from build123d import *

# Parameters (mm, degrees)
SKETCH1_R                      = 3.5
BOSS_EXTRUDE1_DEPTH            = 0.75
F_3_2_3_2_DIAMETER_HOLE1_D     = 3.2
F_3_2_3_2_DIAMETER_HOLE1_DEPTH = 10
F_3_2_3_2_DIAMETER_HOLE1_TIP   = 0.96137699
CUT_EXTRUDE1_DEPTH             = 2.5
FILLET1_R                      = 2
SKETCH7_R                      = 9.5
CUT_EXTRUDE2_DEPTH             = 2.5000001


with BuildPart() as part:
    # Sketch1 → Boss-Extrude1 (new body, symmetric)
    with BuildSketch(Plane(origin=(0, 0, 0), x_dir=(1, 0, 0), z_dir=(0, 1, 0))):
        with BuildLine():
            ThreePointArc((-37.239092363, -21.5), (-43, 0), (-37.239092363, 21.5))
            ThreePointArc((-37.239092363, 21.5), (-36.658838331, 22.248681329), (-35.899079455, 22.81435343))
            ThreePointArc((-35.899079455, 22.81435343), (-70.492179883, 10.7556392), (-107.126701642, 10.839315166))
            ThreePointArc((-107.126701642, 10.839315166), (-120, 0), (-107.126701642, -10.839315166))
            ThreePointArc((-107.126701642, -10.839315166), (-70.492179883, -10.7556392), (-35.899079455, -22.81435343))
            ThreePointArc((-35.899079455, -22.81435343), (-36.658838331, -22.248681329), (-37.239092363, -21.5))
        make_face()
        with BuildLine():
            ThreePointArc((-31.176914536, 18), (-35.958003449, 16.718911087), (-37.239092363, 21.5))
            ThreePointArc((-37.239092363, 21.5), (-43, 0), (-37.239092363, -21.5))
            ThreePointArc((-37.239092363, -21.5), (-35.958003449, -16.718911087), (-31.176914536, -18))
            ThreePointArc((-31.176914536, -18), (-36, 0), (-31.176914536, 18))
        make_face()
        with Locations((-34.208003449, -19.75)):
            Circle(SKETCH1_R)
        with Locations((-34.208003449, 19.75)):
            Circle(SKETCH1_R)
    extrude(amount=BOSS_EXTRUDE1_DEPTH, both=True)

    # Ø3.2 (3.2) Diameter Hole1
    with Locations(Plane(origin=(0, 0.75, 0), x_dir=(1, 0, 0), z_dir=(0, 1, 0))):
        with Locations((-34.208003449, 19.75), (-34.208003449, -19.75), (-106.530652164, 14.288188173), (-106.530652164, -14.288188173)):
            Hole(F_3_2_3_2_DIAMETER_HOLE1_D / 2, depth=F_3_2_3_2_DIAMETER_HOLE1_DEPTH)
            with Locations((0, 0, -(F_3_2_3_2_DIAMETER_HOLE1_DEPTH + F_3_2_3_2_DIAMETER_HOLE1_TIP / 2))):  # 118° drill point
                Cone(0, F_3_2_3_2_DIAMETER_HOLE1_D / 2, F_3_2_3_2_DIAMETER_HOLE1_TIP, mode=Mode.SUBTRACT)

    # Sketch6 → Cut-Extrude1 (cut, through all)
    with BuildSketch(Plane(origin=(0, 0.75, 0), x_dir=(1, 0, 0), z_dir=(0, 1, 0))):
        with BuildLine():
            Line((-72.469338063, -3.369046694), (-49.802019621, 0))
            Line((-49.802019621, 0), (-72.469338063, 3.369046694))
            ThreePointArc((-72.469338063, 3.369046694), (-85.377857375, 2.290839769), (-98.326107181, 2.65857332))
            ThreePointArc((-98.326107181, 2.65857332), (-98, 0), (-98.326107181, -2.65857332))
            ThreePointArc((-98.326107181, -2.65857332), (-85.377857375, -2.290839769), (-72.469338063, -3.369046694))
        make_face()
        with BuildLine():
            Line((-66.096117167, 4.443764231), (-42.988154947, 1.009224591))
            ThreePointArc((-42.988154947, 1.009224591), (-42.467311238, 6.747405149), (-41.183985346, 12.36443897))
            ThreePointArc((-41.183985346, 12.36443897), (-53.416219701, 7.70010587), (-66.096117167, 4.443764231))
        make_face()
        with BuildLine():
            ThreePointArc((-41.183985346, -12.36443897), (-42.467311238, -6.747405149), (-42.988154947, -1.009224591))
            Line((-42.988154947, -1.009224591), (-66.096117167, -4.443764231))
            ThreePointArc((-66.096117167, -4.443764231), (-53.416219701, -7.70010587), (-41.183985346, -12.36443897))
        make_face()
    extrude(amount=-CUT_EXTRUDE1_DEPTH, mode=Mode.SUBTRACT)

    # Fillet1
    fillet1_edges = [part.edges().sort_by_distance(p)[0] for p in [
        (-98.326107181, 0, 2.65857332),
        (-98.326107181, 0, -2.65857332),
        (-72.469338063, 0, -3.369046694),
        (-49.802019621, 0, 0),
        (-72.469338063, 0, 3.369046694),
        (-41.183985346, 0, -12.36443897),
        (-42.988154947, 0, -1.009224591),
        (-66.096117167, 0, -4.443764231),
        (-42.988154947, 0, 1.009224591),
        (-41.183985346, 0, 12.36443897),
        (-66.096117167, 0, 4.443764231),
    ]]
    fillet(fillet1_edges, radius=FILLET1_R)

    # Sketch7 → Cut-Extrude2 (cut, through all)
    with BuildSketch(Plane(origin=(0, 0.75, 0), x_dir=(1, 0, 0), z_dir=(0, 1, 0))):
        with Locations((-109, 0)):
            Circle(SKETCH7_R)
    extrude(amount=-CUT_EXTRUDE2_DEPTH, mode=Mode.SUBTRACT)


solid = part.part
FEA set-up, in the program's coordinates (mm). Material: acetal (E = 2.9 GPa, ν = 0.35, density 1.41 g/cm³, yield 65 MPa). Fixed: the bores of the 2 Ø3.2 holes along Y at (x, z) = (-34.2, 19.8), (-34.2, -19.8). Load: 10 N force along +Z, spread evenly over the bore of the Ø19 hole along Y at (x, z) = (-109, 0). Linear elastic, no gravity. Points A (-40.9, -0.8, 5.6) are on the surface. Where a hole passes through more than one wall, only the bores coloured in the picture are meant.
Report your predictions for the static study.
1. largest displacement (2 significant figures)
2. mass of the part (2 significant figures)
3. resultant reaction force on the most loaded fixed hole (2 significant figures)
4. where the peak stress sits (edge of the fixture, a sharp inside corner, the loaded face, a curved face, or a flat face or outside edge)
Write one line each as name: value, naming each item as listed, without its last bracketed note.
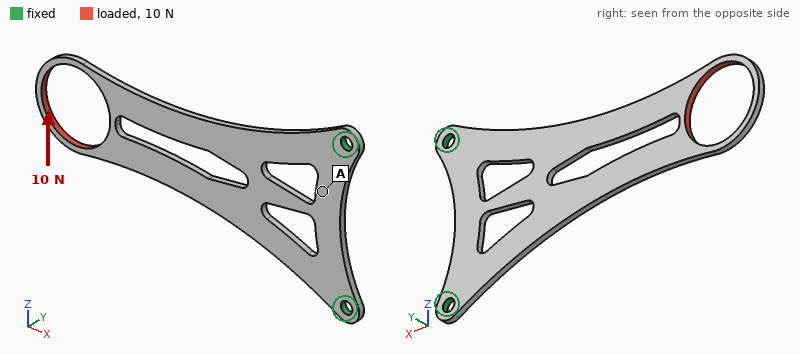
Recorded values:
largest displacement: 1.0 mm
mass of the part: 3.1 g
resultant reaction force on the most loaded fixed hole: 21 N
where the peak stress sits: a curved face
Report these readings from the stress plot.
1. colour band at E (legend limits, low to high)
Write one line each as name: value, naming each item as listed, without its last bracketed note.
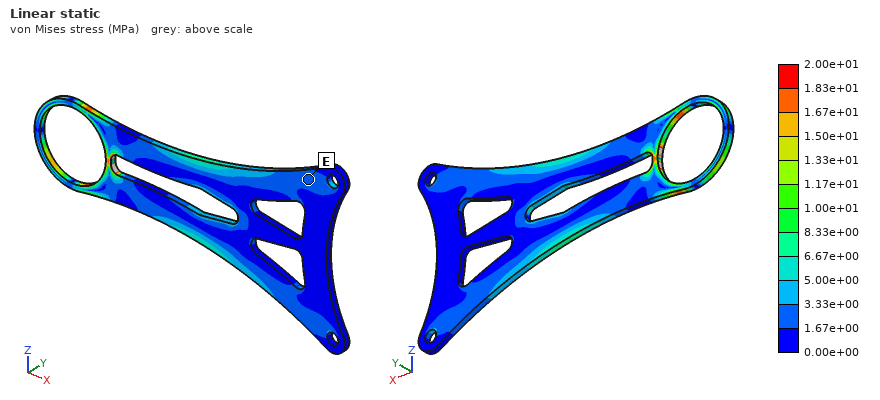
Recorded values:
colour band at E: 1.67e+00 to 3.33e+00 MPa
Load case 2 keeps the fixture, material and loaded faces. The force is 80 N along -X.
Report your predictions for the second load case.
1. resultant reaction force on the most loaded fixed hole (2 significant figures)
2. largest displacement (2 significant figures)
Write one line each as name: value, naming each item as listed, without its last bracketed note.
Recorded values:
resultant reaction force on the most loaded fixed hole: 47 N
largest displacement: 0.72 mm
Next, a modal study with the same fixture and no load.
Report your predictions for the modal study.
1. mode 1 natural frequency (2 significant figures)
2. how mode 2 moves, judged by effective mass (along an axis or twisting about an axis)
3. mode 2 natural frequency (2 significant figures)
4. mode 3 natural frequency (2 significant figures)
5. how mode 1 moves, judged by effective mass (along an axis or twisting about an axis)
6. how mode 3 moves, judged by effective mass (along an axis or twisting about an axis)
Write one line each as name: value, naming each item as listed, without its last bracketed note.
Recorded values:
mode 1 natural frequency: 71 Hz
how mode 2 moves, judged by effective mass: along Y
mode 2 natural frequency: 340 Hz
mode 3 natural frequency: 440 Hz
how mode 1 moves, judged by effective mass: along Y
how mode 3 moves, judged by effective mass: twisting about X
